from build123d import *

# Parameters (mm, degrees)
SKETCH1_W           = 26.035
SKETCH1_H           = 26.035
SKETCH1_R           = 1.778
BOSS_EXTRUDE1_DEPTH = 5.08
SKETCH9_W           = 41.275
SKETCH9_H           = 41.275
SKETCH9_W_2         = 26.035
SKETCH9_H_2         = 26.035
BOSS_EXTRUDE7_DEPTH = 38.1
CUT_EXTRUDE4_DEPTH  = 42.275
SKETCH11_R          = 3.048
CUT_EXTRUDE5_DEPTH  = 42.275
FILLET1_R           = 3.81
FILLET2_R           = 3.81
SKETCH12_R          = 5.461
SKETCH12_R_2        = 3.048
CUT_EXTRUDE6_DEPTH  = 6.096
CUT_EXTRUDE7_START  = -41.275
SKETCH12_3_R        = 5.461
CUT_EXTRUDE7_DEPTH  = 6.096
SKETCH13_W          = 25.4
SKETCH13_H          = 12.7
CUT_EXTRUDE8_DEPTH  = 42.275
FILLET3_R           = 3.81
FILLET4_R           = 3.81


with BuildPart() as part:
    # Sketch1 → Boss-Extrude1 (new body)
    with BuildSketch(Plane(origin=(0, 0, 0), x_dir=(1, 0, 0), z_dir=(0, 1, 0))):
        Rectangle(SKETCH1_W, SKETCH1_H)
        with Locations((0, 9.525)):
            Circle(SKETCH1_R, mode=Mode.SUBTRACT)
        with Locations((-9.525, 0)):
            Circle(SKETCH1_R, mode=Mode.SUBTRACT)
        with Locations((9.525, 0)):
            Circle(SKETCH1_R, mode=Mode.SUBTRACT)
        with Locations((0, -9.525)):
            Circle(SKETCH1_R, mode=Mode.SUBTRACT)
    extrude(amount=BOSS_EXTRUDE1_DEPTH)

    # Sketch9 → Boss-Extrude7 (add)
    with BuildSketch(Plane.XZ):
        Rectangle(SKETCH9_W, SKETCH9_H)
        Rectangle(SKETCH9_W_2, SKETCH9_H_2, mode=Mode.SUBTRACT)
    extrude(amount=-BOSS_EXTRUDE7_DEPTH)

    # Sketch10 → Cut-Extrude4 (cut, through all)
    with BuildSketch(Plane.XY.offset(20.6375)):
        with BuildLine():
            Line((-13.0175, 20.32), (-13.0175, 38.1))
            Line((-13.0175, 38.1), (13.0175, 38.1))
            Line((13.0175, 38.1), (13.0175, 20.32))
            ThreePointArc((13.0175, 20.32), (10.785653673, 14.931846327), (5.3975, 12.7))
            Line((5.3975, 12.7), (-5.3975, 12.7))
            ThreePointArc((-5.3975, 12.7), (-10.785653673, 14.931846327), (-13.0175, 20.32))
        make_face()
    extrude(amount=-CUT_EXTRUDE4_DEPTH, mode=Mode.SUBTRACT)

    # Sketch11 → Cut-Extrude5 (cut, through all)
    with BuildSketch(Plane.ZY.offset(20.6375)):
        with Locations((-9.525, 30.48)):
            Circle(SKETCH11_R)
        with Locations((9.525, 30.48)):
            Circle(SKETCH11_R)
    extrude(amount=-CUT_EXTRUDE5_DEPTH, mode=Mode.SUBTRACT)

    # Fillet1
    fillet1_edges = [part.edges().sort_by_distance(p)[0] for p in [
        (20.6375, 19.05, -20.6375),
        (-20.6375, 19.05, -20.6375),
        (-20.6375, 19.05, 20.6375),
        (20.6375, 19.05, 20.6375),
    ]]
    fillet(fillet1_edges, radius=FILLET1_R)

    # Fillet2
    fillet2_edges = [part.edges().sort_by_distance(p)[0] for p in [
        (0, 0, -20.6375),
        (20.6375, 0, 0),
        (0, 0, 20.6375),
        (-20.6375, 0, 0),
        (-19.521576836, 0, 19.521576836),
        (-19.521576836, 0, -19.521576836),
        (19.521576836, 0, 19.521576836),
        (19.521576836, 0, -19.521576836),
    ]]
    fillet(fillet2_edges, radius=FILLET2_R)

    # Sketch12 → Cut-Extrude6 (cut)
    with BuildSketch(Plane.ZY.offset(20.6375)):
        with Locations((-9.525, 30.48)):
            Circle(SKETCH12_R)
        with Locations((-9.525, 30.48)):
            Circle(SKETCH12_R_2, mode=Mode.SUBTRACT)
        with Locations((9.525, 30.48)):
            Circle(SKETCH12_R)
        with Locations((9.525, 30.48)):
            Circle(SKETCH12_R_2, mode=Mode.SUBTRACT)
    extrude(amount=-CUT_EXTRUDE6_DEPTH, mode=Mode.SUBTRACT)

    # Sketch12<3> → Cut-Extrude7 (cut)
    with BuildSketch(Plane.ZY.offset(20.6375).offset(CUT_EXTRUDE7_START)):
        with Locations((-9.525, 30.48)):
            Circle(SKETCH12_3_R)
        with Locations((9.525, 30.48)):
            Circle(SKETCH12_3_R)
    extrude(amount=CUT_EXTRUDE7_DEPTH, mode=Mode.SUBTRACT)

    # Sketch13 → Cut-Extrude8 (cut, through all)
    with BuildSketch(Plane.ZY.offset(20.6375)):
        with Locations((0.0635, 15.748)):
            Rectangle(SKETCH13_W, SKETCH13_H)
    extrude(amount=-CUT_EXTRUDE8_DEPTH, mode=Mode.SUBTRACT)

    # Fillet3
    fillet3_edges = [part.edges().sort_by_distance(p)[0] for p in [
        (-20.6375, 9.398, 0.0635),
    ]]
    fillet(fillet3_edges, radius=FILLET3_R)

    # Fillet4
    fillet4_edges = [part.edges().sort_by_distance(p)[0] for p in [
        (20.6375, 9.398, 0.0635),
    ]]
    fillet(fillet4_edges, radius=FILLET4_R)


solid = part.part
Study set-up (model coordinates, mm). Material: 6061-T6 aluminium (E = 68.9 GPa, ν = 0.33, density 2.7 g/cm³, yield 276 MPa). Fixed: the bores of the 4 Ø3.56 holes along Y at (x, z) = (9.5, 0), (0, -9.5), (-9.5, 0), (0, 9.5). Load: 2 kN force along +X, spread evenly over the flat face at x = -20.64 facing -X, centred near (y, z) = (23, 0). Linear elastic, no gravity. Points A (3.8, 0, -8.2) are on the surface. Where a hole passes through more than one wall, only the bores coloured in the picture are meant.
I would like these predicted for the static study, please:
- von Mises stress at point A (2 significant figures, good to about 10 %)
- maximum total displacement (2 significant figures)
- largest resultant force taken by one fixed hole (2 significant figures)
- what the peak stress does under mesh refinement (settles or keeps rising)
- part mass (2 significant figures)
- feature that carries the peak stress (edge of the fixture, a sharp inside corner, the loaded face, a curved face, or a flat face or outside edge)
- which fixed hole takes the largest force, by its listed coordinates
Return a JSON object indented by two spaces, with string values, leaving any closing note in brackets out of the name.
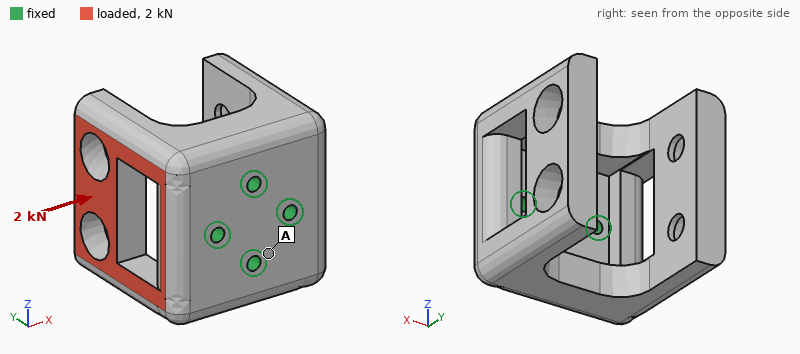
{
  "von Mises stress at point A": "20 MPa",
  "maximum total displacement": "0.24 mm",
  "largest resultant force taken by one fixed hole": "1.7 kN",
  "what the peak stress does under mesh refinement": "keeps rising",
  "part mass": "65 g",
  "feature that carries the peak stress": "edge of the fixture",
  "which fixed hole takes the largest force, by its listed coordinates": "(-9.5, 0)"
}
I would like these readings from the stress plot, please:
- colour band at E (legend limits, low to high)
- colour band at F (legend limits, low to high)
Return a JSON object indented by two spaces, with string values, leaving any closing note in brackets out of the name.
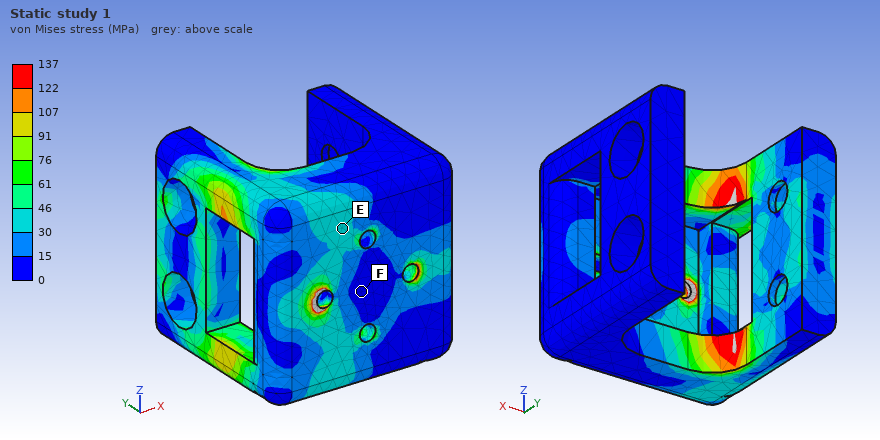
{
  "colour band at E": "30 to 46 MPa",
  "colour band at F": "0 to 15 MPa"
}
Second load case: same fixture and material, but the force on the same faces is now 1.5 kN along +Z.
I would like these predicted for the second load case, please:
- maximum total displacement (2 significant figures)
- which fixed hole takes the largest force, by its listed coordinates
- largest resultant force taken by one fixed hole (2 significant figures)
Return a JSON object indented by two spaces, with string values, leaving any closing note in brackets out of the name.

{
  "maximum total displacement": "0.10 mm",
  "which fixed hole takes the largest force, by its listed coordinates": "(-9.5, 0)",
  "largest resultant force taken by one fixed hole": "1.6 kN"
}
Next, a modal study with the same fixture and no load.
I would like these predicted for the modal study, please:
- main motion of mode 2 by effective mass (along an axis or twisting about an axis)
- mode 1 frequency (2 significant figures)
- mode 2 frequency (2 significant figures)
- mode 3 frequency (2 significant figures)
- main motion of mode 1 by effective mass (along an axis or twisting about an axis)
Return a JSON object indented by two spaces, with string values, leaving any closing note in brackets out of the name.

{
  "main motion of mode 2 by effective mass": "along Z",
  "mode 1 frequency": "4000 Hz",
  "mode 2 frequency": "4600 Hz",
  "mode 3 frequency": "4900 Hz",
  "main motion of mode 1 by effective mass": "along X"
}
